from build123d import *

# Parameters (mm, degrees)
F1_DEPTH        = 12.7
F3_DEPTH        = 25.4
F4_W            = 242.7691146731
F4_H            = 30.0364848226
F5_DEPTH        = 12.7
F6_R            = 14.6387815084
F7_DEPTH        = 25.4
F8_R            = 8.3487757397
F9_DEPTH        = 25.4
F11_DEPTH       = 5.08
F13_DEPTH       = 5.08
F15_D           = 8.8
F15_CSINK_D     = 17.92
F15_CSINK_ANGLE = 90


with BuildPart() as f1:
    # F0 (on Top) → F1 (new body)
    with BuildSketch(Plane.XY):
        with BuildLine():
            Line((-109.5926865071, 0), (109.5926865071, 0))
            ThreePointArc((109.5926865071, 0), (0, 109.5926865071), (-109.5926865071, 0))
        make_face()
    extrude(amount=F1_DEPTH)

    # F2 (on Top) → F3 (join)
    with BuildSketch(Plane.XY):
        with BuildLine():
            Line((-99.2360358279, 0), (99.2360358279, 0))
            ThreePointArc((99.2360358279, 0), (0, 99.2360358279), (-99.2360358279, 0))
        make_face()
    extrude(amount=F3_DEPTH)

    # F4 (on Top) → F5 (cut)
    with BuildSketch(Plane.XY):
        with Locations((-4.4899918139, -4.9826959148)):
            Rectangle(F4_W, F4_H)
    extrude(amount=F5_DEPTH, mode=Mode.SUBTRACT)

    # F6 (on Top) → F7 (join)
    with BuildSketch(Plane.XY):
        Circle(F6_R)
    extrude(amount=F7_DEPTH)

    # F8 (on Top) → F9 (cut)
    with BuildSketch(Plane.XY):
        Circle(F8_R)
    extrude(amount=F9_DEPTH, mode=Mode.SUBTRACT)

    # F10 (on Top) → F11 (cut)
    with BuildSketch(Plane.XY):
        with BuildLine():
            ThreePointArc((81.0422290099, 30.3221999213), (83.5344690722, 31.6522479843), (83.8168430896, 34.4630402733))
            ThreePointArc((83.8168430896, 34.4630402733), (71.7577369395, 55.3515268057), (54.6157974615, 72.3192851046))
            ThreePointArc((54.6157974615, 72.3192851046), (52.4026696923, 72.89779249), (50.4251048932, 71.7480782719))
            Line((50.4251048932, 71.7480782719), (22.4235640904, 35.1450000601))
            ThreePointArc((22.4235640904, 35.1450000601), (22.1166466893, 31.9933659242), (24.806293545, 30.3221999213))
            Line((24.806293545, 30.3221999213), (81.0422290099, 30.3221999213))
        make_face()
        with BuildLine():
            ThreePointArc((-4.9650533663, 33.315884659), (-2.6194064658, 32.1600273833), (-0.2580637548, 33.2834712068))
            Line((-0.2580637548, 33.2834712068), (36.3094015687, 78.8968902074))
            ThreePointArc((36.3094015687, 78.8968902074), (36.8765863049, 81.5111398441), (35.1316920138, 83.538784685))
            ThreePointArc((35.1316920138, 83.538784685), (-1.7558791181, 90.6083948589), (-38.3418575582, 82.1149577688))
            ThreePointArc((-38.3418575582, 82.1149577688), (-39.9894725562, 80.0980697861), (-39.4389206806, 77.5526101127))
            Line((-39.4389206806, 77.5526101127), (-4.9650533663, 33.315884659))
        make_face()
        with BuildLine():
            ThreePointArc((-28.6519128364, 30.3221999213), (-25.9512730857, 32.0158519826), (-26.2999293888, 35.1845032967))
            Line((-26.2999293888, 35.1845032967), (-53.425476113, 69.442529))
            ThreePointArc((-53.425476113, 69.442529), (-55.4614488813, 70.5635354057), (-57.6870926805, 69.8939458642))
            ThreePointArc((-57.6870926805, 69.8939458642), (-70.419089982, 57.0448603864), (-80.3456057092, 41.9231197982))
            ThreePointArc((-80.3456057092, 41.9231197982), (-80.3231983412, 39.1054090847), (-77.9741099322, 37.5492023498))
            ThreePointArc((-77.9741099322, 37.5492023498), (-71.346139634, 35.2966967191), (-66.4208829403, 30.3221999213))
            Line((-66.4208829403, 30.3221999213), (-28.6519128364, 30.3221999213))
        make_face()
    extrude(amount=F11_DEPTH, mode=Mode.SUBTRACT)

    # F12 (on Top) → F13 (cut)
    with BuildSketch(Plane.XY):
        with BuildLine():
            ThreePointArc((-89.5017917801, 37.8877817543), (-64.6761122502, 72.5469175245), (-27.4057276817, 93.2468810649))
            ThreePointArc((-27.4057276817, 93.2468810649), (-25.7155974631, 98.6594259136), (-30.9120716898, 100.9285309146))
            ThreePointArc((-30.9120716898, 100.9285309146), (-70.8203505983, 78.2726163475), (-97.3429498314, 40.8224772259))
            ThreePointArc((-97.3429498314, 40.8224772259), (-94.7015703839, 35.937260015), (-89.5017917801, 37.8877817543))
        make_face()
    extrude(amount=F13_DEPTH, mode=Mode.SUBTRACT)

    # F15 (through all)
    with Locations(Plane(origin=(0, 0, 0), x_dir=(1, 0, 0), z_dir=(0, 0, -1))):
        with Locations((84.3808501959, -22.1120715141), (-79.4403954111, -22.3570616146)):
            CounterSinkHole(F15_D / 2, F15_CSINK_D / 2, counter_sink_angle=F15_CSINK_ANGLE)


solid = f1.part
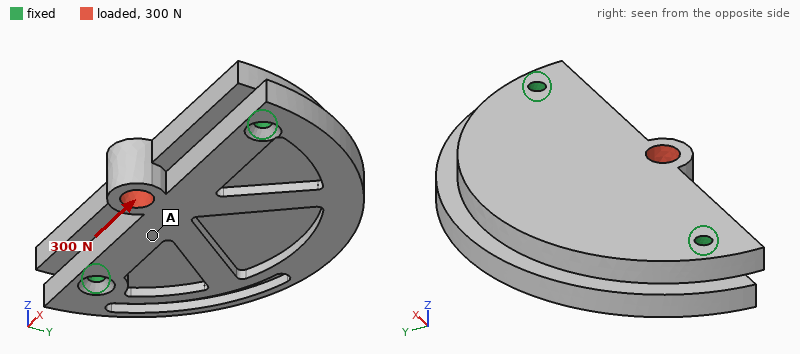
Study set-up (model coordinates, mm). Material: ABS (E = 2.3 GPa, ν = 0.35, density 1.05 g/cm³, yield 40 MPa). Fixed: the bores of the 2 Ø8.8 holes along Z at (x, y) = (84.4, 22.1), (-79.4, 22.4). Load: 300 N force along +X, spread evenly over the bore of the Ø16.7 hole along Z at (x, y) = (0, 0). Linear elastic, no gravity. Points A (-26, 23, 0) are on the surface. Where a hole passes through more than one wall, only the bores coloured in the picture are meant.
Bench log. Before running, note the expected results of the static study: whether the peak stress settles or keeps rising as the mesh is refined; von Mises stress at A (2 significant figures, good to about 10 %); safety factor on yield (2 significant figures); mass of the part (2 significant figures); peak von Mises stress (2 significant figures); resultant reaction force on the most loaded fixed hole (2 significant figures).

settles
0.21 MPa
18
400 g
2.2 MPa
160 N
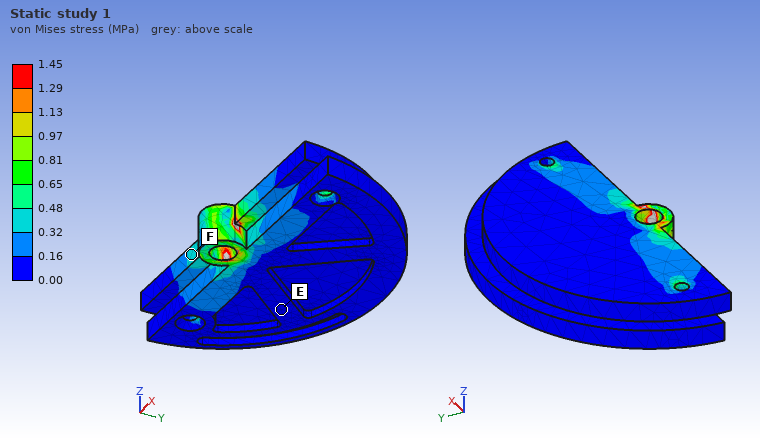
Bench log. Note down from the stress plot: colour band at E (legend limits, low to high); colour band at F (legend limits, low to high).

0.00 to 0.16 MPa
0.32 to 0.48 MPa
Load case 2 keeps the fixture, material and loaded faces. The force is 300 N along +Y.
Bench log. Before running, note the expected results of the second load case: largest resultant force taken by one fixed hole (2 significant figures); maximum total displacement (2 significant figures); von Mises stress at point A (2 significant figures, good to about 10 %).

170 N
31 µm
0.15 MPa
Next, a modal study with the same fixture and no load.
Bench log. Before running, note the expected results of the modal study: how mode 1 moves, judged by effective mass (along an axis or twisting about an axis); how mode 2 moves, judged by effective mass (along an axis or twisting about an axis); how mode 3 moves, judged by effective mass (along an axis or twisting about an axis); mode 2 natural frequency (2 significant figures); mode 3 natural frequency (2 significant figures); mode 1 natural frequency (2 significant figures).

along Z
along Z
twisting about Y
1100 Hz
1400 Hz
510 Hz
